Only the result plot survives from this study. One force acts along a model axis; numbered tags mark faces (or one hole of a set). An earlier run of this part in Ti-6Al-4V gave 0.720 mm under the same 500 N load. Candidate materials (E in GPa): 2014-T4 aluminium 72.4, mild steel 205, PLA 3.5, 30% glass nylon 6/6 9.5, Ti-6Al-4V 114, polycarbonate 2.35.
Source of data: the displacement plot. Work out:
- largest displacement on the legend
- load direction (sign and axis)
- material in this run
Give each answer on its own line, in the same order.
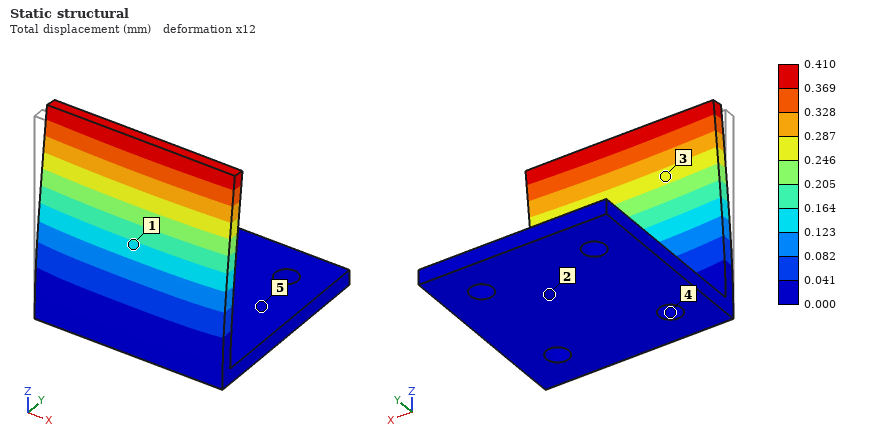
0.410 mm
+Y
mild steel
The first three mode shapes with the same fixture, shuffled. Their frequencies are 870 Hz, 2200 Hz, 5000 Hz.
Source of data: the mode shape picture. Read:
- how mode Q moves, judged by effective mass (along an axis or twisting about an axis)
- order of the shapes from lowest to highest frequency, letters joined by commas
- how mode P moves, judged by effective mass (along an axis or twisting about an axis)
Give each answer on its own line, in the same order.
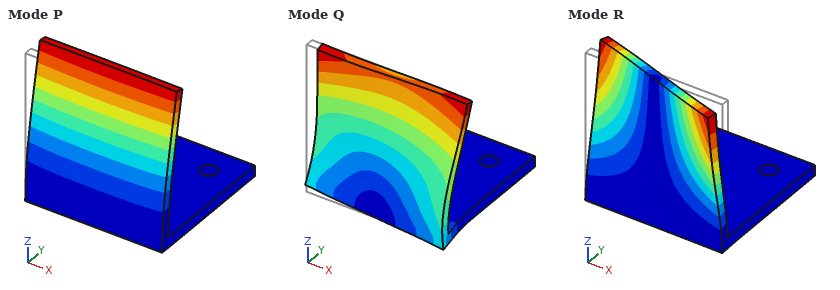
along X
P, R, Q
along Y
